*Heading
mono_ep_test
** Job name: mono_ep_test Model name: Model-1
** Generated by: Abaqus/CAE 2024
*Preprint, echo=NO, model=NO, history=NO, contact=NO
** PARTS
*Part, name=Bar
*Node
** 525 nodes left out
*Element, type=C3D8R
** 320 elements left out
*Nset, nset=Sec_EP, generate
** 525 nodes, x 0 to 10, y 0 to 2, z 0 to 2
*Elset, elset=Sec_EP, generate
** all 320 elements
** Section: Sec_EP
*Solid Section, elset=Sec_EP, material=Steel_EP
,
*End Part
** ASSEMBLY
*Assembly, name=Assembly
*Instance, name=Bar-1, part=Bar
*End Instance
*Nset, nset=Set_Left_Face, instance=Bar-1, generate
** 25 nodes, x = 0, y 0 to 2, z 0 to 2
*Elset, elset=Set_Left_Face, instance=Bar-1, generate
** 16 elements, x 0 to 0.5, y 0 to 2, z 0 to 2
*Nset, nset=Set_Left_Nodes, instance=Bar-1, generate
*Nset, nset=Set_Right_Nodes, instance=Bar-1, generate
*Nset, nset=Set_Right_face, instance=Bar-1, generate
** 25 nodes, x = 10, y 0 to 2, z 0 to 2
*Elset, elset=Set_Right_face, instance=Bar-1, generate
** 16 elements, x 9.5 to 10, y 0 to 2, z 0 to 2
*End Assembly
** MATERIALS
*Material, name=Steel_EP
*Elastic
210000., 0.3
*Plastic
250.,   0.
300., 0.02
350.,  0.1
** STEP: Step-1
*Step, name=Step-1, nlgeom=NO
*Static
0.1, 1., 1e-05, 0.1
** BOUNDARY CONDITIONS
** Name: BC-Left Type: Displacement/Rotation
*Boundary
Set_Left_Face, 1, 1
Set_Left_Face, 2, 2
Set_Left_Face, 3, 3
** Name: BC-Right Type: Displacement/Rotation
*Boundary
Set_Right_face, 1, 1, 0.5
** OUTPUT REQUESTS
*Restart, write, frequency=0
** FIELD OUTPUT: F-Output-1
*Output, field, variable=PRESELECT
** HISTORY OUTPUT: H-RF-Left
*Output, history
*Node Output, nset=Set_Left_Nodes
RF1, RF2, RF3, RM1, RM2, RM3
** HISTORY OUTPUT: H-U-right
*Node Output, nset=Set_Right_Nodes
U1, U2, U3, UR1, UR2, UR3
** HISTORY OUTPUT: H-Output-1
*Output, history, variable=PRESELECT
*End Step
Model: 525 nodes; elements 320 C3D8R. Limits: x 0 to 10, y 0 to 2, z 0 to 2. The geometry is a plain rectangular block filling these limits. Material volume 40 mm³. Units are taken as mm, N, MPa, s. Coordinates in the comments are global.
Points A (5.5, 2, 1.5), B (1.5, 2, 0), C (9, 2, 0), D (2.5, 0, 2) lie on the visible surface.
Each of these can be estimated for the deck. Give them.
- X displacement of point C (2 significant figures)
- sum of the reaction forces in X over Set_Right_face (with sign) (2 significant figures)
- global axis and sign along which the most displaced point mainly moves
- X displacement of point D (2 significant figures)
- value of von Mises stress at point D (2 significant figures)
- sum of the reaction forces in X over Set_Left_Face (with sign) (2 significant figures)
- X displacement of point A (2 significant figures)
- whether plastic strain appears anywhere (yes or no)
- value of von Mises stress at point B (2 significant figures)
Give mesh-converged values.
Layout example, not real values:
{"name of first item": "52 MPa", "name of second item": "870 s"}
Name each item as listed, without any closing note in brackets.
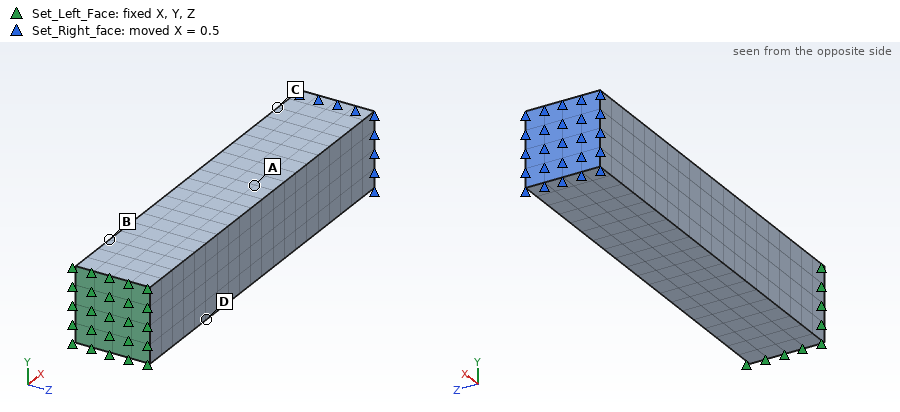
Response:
{"X displacement of point C": "0.45 mm", "sum of the reaction forces in X over Set_Right_face (with sign)": "1300 N", "global axis and sign along which the most displaced point mainly moves": "+X", "X displacement of point D": "0.10 mm", "value of von Mises stress at point D": "320 MPa", "sum of the reaction forces in X over Set_Left_Face (with sign)": "-1300 N", "X displacement of point A": "0.26 mm", "whether plastic strain appears anywhere": "yes", "value of von Mises stress at point B": "310 MPa"}
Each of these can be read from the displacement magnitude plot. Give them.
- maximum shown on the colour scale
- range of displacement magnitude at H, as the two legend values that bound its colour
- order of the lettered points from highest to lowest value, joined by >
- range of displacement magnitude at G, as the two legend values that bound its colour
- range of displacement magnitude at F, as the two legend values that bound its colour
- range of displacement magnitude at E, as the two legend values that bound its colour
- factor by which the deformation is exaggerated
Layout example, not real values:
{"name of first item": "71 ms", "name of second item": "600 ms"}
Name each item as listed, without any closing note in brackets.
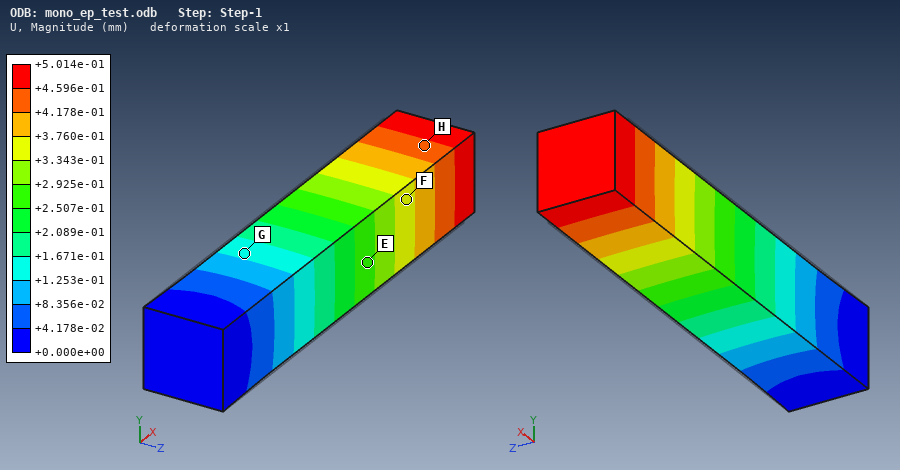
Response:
{"maximum shown on the colour scale": "+5.014e-01 mm", "range of displacement magnitude at H, as the two legend values that bound its colour": "+4.178e-01 to +4.596e-01 mm", "order of the lettered points from highest to lowest value, joined by >": "H > F > E > G", "range of displacement magnitude at G, as the two legend values that bound its colour": "+1.253e-01 to +1.671e-01 mm", "range of displacement magnitude at F, as the two legend values that bound its colour": "+3.343e-01 to +3.760e-01 mm", "range of displacement magnitude at E, as the two legend values that bound its colour": "+2.507e-01 to +2.925e-01 mm", "factor by which the deformation is exaggerated": "1"}
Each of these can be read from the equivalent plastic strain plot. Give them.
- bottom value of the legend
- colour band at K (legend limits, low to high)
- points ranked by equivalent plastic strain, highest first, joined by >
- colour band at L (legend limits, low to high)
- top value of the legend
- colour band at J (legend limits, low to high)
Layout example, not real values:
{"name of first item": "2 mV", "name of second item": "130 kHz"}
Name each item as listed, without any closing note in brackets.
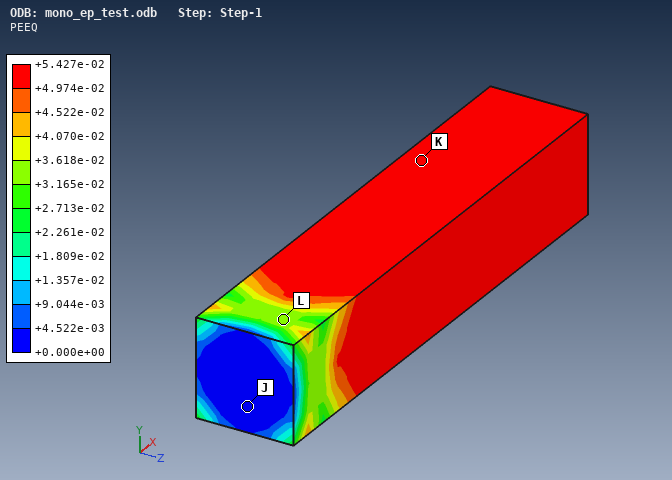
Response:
{"bottom value of the legend": "+0.000e+00", "colour band at K": "+4.974e-02 to +5.427e-02", "points ranked by equivalent plastic strain, highest first, joined by >": "K > L > J", "colour band at L": "+3.165e-02 to +3.618e-02", "top value of the legend": "+5.427e-02", "colour band at J": "+0.000e+00 to +4.522e-03"}
